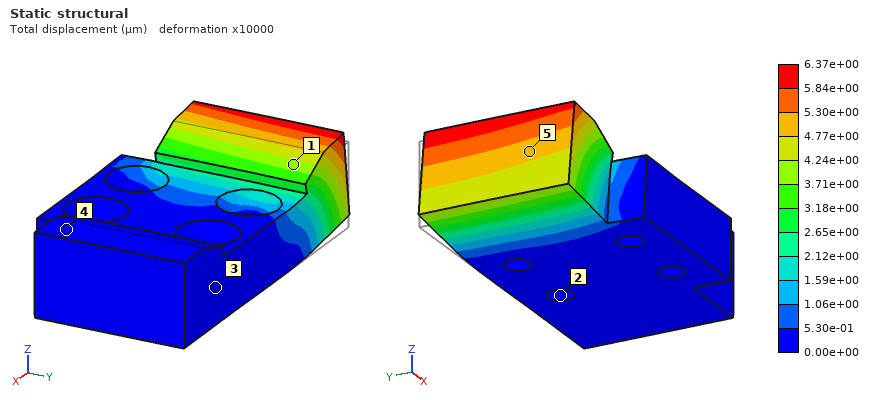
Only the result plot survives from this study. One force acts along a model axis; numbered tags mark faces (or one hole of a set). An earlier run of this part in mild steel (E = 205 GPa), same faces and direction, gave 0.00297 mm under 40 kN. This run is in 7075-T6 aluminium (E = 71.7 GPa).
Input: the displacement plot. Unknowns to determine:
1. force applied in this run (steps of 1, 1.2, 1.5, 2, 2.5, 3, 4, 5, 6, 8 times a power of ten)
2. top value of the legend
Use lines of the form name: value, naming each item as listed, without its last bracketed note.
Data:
force applied in this run: 30 kN
top value of the legend: 6.37e+00 µm
